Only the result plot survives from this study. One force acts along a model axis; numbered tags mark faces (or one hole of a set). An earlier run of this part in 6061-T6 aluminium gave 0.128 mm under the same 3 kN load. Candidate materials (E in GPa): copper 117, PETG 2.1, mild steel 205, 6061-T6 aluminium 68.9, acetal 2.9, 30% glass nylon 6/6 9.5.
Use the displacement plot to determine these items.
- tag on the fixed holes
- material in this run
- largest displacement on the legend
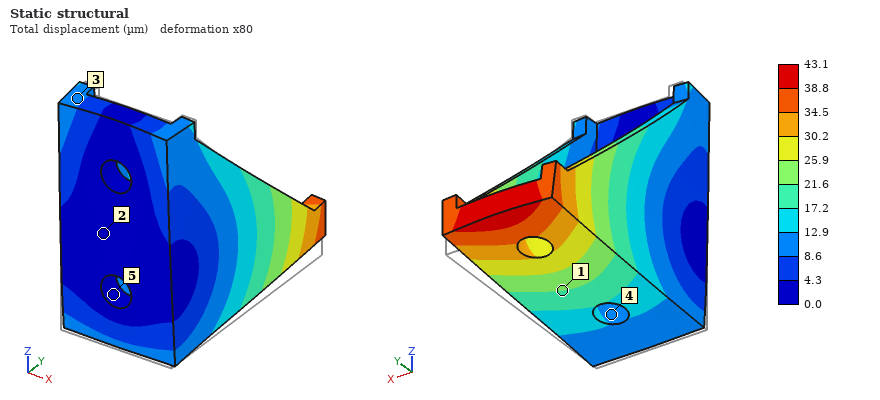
5
mild steel
43.1 µm
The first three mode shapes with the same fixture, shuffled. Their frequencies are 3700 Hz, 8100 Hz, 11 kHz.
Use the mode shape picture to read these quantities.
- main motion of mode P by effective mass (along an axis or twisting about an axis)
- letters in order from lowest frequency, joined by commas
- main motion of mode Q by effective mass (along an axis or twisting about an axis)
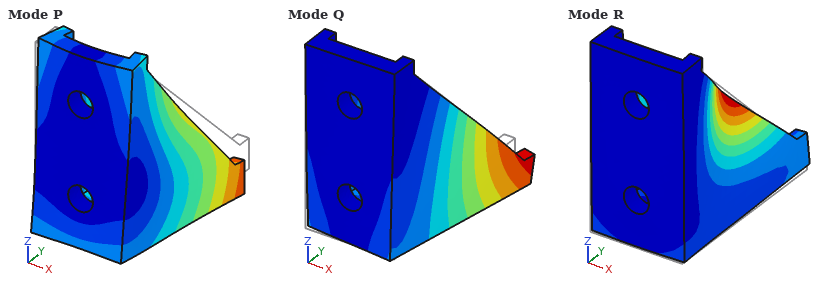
along Z
Q, P, R
along X
